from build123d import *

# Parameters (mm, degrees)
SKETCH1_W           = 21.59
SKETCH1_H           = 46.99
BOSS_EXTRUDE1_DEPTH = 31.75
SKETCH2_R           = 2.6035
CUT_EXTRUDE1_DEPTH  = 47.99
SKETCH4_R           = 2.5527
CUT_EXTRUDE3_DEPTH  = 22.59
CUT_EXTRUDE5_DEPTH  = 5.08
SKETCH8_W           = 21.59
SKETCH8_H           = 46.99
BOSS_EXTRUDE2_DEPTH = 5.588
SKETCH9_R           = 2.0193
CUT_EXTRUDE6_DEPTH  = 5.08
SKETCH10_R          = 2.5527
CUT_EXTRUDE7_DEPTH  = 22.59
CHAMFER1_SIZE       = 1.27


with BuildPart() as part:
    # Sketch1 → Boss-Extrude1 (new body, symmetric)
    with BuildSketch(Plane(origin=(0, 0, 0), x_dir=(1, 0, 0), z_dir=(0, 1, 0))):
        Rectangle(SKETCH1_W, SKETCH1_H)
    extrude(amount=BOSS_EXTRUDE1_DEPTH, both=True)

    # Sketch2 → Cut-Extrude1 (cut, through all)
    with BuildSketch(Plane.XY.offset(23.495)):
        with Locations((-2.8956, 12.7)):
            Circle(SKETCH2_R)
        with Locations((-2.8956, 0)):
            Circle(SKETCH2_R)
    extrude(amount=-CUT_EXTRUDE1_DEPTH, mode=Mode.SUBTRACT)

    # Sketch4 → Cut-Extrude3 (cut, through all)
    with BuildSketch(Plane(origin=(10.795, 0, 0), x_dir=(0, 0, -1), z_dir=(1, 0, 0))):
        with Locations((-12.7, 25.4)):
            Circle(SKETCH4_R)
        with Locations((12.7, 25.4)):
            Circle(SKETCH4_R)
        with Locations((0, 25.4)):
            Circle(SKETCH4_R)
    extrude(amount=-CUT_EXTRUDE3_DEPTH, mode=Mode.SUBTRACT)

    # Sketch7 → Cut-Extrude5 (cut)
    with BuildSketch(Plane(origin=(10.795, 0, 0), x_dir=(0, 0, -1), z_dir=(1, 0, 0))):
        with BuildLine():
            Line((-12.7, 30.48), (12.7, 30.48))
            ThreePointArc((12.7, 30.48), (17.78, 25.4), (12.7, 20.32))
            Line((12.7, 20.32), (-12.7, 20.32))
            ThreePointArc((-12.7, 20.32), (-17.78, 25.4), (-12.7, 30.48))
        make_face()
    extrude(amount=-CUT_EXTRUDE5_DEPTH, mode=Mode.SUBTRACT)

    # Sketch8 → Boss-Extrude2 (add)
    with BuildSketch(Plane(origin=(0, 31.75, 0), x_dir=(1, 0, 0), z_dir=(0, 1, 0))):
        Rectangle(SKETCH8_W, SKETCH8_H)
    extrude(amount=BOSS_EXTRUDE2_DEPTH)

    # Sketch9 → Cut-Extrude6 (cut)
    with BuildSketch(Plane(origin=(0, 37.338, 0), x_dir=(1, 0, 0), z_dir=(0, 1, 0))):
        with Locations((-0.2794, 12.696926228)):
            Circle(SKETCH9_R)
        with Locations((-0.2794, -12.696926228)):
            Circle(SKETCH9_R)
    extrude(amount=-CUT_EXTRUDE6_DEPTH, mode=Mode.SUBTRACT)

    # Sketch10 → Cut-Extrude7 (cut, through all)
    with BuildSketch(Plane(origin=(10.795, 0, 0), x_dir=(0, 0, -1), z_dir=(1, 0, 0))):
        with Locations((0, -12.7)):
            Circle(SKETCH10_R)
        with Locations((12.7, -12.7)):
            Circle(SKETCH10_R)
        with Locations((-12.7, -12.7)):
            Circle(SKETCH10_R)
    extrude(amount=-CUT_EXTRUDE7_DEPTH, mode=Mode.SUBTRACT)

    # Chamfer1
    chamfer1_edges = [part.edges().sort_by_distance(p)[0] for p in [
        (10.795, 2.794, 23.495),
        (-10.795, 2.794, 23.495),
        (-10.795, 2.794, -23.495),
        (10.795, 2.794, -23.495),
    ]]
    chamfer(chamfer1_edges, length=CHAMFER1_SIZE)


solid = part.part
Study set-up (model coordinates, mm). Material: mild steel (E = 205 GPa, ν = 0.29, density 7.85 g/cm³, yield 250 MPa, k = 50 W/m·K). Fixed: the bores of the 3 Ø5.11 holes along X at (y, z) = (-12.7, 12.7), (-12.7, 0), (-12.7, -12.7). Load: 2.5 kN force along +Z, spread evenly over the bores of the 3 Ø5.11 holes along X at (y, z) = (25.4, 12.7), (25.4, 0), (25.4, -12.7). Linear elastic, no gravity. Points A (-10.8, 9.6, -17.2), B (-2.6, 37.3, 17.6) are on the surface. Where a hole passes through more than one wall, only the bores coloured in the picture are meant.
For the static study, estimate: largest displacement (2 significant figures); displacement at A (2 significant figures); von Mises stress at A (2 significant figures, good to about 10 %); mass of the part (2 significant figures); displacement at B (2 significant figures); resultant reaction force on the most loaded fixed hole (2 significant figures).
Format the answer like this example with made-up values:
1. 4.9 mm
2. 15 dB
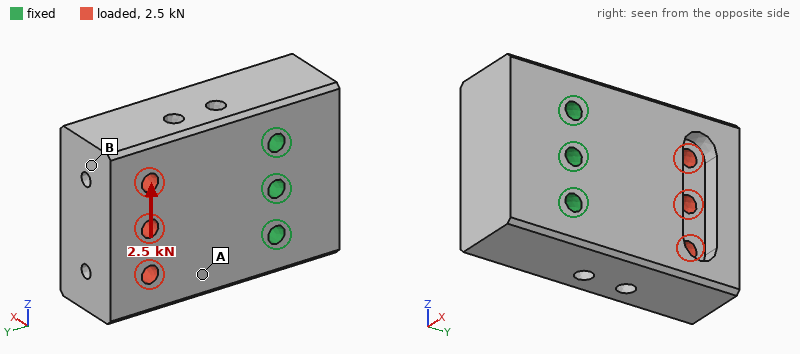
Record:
1. 5.1 µm
2. 2.2 µm
3. 6.8 MPa
4. 500 g
5. 4.8 µm
6. 3.4 kN
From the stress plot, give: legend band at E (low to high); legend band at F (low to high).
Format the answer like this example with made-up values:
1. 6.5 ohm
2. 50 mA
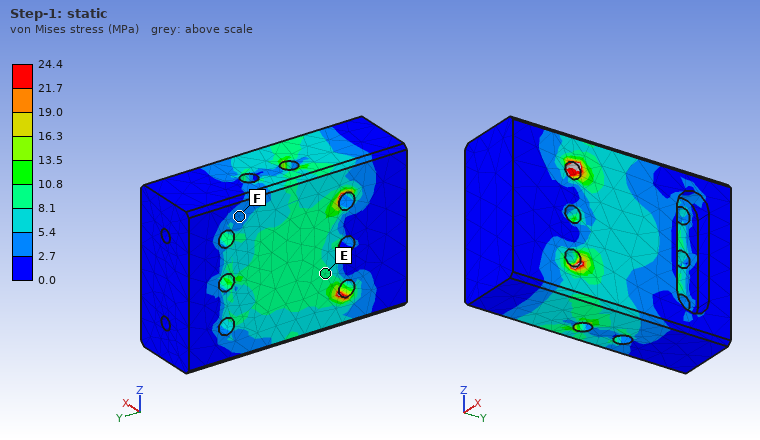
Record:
1. 8.1 to 10.8 MPa
2. 2.7 to 5.4 MPa
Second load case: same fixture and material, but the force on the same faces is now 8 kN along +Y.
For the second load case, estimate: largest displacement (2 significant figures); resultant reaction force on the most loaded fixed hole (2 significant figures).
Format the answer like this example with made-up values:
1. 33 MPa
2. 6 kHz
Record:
1. 4.7 µm
2. 3.0 kN
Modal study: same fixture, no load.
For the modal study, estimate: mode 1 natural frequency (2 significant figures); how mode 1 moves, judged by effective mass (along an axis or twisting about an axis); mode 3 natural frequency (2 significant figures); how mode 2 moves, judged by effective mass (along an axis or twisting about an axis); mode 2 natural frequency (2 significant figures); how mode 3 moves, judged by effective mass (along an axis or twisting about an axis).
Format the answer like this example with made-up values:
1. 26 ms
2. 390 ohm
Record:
1. 6400 Hz
2. along X
3. 12 kHz
4. along Z
5. 9200 Hz
6. twisting about Y
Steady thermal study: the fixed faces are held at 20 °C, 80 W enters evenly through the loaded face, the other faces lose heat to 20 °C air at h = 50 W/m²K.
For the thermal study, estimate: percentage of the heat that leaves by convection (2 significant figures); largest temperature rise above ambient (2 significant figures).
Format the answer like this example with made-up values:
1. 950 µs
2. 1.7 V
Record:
1. 22 %
2. 65 K
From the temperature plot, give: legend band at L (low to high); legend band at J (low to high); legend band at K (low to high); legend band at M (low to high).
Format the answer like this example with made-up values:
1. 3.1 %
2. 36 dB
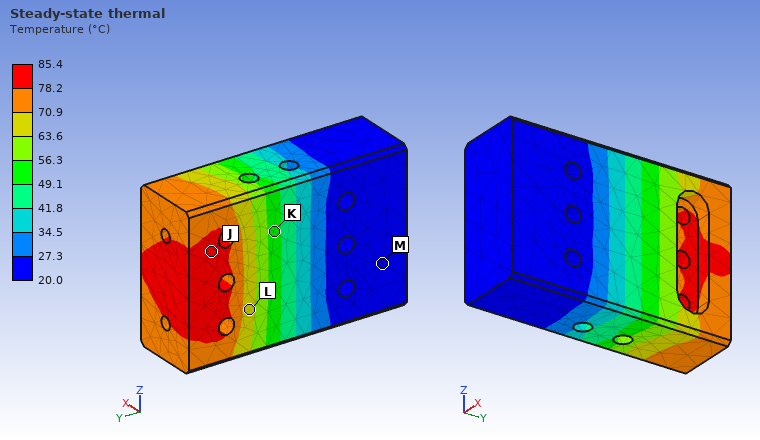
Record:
1. 63.6 to 70.9 °C
2. 78.2 to 85.4 °C
3. 49.1 to 56.3 °C
4. 20.0 to 27.3 °C
